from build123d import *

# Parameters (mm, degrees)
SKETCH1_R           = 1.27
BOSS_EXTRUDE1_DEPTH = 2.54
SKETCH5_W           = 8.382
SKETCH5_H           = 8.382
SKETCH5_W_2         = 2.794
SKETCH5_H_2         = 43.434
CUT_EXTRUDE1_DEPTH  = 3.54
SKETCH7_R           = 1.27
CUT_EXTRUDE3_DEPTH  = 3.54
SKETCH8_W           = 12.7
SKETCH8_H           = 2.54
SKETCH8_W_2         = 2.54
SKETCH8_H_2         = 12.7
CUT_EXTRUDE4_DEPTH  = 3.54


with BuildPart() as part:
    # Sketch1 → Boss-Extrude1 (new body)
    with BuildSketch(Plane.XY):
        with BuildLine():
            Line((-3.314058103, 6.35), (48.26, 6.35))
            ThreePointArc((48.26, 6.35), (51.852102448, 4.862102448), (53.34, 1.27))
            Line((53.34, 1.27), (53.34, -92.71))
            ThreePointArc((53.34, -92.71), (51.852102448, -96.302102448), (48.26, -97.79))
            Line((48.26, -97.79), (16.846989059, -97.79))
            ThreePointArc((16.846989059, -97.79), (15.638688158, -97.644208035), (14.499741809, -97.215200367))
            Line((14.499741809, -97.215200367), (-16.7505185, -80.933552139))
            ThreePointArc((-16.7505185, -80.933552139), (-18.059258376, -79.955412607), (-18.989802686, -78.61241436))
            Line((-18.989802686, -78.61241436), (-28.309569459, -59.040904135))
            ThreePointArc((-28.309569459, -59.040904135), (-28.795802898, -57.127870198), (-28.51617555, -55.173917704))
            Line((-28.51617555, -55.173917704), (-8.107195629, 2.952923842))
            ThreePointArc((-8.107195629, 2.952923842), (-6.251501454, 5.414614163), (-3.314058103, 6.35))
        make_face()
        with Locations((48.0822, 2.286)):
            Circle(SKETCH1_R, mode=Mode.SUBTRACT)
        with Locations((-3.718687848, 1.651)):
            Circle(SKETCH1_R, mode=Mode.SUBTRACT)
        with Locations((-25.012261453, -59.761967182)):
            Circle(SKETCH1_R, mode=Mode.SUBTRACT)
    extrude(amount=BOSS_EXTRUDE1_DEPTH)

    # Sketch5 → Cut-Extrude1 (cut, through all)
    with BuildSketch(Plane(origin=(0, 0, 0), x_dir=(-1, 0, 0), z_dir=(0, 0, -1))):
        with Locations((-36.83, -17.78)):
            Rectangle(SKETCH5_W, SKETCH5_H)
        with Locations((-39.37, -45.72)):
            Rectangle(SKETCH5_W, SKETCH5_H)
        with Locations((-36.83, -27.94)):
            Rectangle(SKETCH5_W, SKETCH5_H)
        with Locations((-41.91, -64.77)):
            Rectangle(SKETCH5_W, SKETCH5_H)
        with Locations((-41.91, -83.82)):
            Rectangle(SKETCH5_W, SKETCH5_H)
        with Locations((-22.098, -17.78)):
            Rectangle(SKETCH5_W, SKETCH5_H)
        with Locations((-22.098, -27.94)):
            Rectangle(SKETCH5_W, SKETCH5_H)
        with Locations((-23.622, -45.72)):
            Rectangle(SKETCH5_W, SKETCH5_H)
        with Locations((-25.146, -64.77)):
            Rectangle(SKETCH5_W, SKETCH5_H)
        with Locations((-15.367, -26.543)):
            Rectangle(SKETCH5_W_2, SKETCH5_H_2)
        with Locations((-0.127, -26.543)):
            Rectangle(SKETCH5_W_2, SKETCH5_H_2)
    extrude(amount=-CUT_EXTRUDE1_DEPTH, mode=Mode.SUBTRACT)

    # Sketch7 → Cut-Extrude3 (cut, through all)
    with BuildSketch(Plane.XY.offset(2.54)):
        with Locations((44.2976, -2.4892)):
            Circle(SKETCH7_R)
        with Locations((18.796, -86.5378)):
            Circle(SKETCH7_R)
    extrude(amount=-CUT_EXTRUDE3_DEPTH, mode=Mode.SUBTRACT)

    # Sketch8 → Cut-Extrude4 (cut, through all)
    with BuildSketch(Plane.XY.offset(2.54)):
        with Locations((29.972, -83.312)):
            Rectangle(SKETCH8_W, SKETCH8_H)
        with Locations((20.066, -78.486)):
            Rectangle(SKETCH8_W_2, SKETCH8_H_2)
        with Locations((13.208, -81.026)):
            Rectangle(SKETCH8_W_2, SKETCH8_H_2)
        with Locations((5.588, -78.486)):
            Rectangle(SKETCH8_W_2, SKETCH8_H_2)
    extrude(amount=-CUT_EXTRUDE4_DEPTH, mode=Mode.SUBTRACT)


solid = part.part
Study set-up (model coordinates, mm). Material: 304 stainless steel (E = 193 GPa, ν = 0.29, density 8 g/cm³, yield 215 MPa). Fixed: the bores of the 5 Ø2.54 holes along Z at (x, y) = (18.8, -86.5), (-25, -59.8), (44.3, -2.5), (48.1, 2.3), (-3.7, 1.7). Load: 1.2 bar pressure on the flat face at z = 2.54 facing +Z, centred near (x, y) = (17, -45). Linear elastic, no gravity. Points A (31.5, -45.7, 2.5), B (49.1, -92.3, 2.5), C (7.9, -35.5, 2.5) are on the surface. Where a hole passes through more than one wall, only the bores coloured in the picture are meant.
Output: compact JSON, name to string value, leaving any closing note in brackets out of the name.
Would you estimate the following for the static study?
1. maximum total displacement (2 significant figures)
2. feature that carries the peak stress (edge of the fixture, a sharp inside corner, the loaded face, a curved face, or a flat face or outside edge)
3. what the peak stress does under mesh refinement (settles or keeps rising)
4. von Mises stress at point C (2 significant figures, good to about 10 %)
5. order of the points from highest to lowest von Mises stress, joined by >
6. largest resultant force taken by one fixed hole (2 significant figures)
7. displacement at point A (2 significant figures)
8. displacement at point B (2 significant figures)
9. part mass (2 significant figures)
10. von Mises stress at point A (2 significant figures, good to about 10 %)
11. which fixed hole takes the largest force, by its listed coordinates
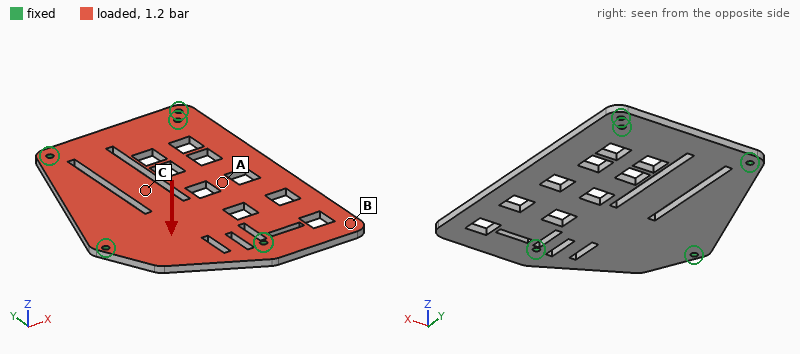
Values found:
{"maximum total displacement": "0.18 mm", "feature that carries the peak stress": "edge of the fixture", "what the peak stress does under mesh refinement": "keeps rising", "von Mises stress at point C": "33 MPa", "order of the points from highest to lowest von Mises stress, joined by >": "A > C > B", "largest resultant force taken by one fixed hole": "340 N", "displacement at point A": "0.12 mm", "displacement at point B": "0.11 mm", "part mass": "130 g", "von Mises stress at point A": "58 MPa", "which fixed hole takes the largest force, by its listed coordinates": "(44.3, -2.5)"}
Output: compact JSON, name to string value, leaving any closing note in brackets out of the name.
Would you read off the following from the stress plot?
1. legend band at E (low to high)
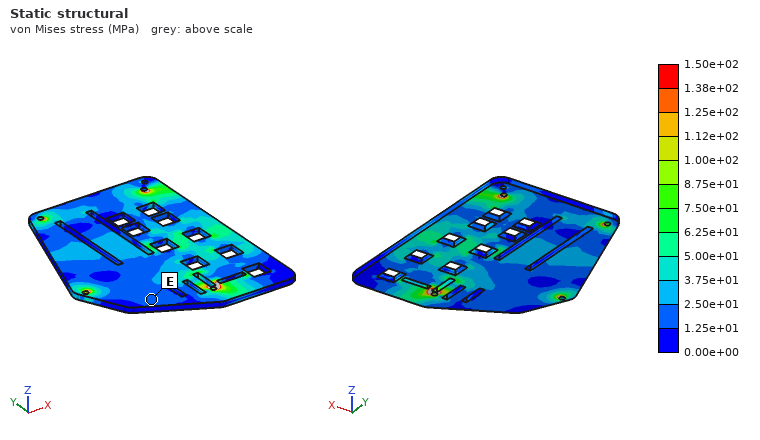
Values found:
{"legend band at E": "1.25e+01 to 2.50e+01 MPa"}
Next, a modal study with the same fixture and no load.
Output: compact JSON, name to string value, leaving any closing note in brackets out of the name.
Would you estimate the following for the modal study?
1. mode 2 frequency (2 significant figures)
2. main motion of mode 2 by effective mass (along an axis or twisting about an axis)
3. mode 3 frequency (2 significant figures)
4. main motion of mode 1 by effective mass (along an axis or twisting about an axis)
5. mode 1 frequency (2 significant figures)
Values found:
{"mode 2 frequency": "1800 Hz", "main motion of mode 2 by effective mass": "along Z", "mode 3 frequency": "2600 Hz", "main motion of mode 1 by effective mass": "along Z", "mode 1 frequency": "1200 Hz"}
